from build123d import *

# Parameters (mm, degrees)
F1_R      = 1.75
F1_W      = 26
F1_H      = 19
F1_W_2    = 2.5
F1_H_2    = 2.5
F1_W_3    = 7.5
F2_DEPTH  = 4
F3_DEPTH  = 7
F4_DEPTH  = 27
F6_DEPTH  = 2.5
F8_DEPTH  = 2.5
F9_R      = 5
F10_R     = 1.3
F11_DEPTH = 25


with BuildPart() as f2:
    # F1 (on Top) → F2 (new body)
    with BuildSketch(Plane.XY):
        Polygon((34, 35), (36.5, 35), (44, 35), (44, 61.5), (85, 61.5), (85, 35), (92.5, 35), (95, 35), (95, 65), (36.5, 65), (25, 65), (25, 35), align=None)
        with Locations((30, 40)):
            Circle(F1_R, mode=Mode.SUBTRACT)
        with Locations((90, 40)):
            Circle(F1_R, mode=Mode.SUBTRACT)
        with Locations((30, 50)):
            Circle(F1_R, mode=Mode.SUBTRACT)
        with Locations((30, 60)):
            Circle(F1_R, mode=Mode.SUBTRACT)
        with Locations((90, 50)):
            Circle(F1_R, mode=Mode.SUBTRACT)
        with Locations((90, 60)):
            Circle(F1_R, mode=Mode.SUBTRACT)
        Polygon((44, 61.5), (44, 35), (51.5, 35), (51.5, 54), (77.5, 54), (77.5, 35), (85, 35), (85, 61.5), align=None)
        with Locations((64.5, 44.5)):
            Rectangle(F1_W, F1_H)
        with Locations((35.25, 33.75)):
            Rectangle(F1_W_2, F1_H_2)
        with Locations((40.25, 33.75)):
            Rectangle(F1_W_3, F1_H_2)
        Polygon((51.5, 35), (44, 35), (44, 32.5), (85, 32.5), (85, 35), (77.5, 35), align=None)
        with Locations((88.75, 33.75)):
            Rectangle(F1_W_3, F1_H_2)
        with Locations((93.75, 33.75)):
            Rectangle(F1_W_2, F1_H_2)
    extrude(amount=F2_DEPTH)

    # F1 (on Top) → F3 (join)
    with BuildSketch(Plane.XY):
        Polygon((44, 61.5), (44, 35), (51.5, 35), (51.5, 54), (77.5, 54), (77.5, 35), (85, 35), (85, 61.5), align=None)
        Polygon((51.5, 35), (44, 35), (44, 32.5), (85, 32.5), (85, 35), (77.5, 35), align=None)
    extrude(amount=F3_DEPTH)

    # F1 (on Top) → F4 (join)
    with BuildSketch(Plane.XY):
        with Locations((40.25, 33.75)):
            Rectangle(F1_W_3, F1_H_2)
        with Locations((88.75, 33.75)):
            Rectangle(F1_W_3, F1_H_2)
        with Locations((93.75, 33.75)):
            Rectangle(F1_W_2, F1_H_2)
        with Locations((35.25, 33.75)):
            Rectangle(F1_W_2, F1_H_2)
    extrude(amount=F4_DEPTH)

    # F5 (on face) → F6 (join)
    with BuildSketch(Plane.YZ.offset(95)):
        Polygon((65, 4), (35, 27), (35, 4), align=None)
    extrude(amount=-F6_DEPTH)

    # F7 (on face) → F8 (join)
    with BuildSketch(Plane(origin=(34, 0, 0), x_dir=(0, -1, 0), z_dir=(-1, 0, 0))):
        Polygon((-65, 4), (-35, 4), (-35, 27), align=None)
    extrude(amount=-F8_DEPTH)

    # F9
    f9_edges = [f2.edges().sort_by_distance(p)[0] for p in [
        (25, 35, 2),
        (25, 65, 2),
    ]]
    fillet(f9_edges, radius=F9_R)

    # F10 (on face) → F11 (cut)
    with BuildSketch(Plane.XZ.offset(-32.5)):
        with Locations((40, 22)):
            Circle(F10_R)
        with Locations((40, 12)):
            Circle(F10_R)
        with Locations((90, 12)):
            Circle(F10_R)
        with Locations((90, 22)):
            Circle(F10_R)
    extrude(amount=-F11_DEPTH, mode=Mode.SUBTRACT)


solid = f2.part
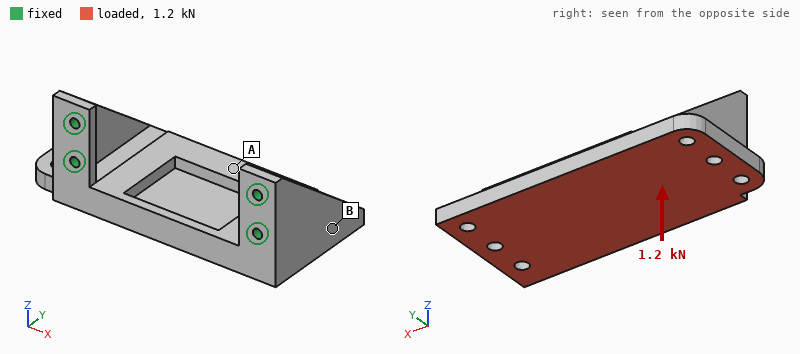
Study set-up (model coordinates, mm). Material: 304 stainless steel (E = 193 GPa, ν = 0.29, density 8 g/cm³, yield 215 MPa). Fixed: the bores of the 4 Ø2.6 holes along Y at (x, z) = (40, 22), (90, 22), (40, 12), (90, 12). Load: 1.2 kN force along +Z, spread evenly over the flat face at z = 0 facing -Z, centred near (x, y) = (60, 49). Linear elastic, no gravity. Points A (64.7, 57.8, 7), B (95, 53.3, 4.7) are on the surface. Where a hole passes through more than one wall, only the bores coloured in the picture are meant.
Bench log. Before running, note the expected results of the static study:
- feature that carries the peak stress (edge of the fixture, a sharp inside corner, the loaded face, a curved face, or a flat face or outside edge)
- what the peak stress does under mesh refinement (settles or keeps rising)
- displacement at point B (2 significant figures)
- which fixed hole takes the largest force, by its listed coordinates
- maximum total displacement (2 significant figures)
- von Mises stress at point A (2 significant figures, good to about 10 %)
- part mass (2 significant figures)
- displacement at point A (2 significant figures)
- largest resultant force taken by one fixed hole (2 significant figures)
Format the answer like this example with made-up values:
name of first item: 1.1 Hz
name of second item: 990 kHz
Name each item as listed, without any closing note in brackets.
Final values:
feature that carries the peak stress: edge of the fixture
what the peak stress does under mesh refinement: keeps rising
displacement at point B: 20 µm
which fixed hole takes the largest force, by its listed coordinates: (40, 12)
maximum total displacement: 66 µm
von Mises stress at point A: 38 MPa
part mass: 110 g
displacement at point A: 50 µm
largest resultant force taken by one fixed hole: 940 N
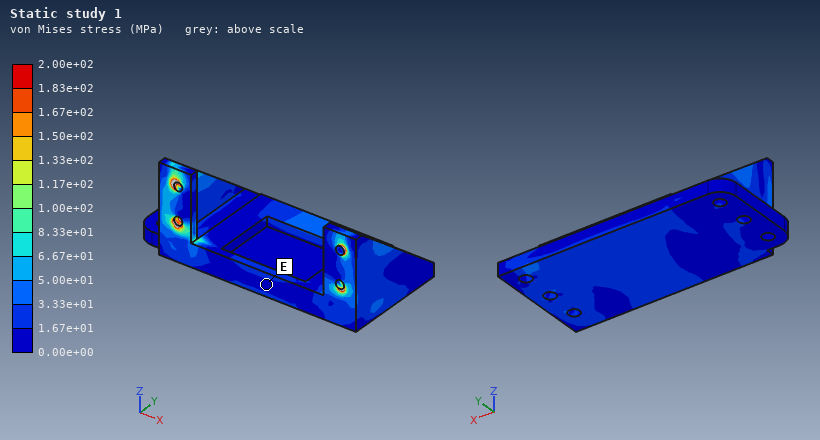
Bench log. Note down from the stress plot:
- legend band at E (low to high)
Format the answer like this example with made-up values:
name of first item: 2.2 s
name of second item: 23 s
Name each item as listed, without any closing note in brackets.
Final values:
legend band at E: 0.00e+00 to 1.67e+01 MPa
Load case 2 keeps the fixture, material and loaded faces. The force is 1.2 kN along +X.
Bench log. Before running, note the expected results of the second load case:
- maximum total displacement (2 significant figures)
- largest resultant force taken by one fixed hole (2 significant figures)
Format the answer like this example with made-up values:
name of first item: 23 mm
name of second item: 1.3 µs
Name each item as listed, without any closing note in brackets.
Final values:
maximum total displacement: 18 µm
largest resultant force taken by one fixed hole: 870 N
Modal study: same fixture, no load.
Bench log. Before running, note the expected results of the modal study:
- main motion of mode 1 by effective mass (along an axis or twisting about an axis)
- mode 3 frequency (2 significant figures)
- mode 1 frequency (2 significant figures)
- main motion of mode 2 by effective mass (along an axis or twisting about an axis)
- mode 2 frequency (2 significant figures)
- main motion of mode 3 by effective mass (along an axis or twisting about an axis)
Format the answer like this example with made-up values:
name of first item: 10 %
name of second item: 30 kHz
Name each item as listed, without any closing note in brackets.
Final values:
main motion of mode 1 by effective mass: along Z
mode 3 frequency: 6600 Hz
mode 1 frequency: 2700 Hz
main motion of mode 2 by effective mass: along X
mode 2 frequency: 4200 Hz
main motion of mode 3 by effective mass: along Y
